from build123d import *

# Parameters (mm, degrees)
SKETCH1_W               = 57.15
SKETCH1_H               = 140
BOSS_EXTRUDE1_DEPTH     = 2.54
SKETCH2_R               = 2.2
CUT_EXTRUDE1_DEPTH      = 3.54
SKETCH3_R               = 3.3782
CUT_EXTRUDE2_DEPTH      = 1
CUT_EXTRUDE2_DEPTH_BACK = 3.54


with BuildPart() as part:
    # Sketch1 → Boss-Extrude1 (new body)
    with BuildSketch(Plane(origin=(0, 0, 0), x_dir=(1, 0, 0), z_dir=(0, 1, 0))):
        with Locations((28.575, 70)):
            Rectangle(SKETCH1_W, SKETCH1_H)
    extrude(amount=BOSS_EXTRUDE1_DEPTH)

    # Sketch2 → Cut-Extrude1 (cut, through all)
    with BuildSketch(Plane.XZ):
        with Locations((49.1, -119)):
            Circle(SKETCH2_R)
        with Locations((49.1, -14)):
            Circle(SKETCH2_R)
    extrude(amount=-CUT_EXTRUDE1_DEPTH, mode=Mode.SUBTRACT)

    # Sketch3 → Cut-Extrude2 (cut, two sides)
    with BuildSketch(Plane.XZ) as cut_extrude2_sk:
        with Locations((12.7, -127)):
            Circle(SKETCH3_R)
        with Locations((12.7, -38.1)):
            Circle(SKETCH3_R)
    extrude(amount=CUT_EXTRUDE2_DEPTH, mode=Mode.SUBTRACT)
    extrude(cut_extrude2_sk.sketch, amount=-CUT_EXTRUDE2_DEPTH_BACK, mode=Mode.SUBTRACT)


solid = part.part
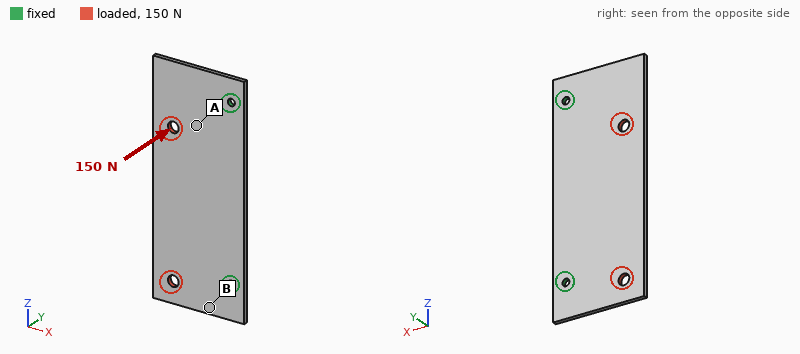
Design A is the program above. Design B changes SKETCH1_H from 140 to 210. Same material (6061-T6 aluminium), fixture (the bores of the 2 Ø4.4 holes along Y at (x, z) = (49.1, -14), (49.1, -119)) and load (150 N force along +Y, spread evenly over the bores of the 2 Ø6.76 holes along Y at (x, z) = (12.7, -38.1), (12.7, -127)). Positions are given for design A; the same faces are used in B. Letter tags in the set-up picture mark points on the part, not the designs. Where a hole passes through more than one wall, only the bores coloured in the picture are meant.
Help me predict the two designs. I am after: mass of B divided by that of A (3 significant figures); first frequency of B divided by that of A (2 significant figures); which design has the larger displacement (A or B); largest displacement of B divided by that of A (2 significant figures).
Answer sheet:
1.51
0.84
A
0.89
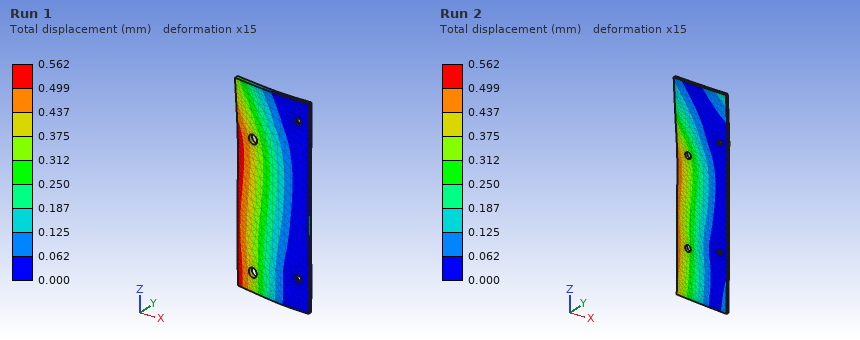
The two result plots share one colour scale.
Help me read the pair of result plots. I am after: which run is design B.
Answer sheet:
Run 2
